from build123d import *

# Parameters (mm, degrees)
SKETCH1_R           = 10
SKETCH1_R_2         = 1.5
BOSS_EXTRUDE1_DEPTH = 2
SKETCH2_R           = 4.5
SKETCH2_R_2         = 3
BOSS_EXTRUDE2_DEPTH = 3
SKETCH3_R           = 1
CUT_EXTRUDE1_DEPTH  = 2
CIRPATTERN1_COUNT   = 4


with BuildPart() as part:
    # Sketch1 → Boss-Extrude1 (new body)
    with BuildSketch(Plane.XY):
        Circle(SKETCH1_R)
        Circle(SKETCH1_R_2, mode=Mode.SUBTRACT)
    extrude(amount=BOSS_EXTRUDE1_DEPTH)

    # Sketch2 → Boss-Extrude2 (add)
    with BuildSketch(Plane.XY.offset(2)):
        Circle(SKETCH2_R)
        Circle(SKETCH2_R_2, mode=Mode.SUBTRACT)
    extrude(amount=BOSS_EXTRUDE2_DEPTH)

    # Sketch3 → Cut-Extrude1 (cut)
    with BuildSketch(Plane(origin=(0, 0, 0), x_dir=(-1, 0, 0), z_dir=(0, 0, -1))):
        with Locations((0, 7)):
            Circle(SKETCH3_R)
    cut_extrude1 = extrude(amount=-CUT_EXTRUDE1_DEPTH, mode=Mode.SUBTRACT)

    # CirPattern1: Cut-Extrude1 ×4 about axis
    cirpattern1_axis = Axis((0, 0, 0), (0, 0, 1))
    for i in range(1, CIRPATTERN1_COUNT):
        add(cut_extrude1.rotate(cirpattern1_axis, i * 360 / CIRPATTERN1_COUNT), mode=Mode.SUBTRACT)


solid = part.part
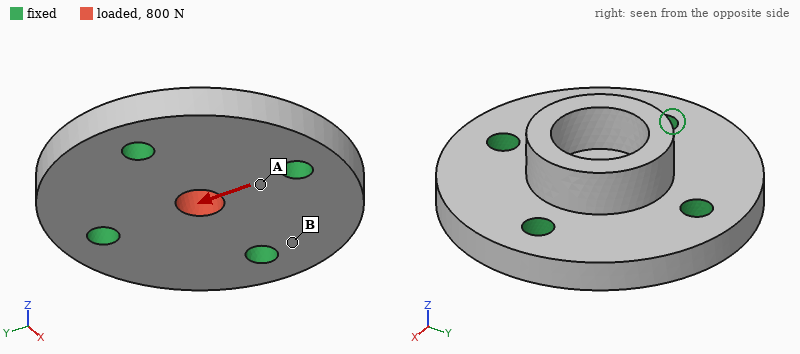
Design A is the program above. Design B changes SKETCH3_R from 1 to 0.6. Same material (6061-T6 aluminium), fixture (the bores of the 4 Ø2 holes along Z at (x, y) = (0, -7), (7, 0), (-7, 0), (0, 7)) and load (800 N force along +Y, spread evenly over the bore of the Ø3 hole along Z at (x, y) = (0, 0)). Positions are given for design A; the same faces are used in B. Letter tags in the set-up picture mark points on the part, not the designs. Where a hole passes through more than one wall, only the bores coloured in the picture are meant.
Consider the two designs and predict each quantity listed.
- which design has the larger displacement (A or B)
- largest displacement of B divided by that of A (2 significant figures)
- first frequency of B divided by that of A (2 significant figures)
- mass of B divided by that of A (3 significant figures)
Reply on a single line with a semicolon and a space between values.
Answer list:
B; 1.1; 0.82; 1.02
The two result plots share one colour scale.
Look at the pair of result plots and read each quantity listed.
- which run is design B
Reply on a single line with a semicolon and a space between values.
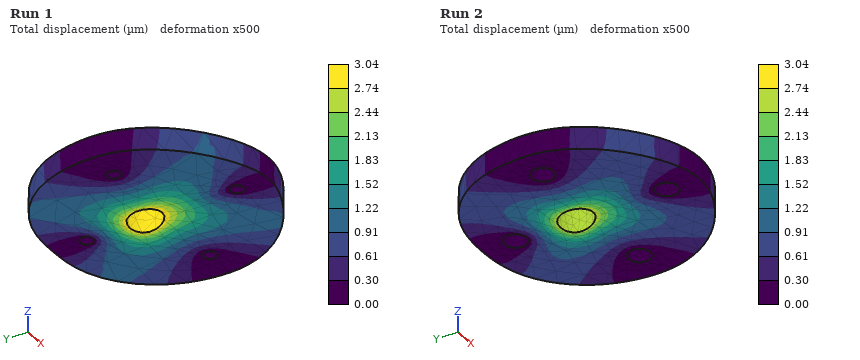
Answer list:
Run 1
